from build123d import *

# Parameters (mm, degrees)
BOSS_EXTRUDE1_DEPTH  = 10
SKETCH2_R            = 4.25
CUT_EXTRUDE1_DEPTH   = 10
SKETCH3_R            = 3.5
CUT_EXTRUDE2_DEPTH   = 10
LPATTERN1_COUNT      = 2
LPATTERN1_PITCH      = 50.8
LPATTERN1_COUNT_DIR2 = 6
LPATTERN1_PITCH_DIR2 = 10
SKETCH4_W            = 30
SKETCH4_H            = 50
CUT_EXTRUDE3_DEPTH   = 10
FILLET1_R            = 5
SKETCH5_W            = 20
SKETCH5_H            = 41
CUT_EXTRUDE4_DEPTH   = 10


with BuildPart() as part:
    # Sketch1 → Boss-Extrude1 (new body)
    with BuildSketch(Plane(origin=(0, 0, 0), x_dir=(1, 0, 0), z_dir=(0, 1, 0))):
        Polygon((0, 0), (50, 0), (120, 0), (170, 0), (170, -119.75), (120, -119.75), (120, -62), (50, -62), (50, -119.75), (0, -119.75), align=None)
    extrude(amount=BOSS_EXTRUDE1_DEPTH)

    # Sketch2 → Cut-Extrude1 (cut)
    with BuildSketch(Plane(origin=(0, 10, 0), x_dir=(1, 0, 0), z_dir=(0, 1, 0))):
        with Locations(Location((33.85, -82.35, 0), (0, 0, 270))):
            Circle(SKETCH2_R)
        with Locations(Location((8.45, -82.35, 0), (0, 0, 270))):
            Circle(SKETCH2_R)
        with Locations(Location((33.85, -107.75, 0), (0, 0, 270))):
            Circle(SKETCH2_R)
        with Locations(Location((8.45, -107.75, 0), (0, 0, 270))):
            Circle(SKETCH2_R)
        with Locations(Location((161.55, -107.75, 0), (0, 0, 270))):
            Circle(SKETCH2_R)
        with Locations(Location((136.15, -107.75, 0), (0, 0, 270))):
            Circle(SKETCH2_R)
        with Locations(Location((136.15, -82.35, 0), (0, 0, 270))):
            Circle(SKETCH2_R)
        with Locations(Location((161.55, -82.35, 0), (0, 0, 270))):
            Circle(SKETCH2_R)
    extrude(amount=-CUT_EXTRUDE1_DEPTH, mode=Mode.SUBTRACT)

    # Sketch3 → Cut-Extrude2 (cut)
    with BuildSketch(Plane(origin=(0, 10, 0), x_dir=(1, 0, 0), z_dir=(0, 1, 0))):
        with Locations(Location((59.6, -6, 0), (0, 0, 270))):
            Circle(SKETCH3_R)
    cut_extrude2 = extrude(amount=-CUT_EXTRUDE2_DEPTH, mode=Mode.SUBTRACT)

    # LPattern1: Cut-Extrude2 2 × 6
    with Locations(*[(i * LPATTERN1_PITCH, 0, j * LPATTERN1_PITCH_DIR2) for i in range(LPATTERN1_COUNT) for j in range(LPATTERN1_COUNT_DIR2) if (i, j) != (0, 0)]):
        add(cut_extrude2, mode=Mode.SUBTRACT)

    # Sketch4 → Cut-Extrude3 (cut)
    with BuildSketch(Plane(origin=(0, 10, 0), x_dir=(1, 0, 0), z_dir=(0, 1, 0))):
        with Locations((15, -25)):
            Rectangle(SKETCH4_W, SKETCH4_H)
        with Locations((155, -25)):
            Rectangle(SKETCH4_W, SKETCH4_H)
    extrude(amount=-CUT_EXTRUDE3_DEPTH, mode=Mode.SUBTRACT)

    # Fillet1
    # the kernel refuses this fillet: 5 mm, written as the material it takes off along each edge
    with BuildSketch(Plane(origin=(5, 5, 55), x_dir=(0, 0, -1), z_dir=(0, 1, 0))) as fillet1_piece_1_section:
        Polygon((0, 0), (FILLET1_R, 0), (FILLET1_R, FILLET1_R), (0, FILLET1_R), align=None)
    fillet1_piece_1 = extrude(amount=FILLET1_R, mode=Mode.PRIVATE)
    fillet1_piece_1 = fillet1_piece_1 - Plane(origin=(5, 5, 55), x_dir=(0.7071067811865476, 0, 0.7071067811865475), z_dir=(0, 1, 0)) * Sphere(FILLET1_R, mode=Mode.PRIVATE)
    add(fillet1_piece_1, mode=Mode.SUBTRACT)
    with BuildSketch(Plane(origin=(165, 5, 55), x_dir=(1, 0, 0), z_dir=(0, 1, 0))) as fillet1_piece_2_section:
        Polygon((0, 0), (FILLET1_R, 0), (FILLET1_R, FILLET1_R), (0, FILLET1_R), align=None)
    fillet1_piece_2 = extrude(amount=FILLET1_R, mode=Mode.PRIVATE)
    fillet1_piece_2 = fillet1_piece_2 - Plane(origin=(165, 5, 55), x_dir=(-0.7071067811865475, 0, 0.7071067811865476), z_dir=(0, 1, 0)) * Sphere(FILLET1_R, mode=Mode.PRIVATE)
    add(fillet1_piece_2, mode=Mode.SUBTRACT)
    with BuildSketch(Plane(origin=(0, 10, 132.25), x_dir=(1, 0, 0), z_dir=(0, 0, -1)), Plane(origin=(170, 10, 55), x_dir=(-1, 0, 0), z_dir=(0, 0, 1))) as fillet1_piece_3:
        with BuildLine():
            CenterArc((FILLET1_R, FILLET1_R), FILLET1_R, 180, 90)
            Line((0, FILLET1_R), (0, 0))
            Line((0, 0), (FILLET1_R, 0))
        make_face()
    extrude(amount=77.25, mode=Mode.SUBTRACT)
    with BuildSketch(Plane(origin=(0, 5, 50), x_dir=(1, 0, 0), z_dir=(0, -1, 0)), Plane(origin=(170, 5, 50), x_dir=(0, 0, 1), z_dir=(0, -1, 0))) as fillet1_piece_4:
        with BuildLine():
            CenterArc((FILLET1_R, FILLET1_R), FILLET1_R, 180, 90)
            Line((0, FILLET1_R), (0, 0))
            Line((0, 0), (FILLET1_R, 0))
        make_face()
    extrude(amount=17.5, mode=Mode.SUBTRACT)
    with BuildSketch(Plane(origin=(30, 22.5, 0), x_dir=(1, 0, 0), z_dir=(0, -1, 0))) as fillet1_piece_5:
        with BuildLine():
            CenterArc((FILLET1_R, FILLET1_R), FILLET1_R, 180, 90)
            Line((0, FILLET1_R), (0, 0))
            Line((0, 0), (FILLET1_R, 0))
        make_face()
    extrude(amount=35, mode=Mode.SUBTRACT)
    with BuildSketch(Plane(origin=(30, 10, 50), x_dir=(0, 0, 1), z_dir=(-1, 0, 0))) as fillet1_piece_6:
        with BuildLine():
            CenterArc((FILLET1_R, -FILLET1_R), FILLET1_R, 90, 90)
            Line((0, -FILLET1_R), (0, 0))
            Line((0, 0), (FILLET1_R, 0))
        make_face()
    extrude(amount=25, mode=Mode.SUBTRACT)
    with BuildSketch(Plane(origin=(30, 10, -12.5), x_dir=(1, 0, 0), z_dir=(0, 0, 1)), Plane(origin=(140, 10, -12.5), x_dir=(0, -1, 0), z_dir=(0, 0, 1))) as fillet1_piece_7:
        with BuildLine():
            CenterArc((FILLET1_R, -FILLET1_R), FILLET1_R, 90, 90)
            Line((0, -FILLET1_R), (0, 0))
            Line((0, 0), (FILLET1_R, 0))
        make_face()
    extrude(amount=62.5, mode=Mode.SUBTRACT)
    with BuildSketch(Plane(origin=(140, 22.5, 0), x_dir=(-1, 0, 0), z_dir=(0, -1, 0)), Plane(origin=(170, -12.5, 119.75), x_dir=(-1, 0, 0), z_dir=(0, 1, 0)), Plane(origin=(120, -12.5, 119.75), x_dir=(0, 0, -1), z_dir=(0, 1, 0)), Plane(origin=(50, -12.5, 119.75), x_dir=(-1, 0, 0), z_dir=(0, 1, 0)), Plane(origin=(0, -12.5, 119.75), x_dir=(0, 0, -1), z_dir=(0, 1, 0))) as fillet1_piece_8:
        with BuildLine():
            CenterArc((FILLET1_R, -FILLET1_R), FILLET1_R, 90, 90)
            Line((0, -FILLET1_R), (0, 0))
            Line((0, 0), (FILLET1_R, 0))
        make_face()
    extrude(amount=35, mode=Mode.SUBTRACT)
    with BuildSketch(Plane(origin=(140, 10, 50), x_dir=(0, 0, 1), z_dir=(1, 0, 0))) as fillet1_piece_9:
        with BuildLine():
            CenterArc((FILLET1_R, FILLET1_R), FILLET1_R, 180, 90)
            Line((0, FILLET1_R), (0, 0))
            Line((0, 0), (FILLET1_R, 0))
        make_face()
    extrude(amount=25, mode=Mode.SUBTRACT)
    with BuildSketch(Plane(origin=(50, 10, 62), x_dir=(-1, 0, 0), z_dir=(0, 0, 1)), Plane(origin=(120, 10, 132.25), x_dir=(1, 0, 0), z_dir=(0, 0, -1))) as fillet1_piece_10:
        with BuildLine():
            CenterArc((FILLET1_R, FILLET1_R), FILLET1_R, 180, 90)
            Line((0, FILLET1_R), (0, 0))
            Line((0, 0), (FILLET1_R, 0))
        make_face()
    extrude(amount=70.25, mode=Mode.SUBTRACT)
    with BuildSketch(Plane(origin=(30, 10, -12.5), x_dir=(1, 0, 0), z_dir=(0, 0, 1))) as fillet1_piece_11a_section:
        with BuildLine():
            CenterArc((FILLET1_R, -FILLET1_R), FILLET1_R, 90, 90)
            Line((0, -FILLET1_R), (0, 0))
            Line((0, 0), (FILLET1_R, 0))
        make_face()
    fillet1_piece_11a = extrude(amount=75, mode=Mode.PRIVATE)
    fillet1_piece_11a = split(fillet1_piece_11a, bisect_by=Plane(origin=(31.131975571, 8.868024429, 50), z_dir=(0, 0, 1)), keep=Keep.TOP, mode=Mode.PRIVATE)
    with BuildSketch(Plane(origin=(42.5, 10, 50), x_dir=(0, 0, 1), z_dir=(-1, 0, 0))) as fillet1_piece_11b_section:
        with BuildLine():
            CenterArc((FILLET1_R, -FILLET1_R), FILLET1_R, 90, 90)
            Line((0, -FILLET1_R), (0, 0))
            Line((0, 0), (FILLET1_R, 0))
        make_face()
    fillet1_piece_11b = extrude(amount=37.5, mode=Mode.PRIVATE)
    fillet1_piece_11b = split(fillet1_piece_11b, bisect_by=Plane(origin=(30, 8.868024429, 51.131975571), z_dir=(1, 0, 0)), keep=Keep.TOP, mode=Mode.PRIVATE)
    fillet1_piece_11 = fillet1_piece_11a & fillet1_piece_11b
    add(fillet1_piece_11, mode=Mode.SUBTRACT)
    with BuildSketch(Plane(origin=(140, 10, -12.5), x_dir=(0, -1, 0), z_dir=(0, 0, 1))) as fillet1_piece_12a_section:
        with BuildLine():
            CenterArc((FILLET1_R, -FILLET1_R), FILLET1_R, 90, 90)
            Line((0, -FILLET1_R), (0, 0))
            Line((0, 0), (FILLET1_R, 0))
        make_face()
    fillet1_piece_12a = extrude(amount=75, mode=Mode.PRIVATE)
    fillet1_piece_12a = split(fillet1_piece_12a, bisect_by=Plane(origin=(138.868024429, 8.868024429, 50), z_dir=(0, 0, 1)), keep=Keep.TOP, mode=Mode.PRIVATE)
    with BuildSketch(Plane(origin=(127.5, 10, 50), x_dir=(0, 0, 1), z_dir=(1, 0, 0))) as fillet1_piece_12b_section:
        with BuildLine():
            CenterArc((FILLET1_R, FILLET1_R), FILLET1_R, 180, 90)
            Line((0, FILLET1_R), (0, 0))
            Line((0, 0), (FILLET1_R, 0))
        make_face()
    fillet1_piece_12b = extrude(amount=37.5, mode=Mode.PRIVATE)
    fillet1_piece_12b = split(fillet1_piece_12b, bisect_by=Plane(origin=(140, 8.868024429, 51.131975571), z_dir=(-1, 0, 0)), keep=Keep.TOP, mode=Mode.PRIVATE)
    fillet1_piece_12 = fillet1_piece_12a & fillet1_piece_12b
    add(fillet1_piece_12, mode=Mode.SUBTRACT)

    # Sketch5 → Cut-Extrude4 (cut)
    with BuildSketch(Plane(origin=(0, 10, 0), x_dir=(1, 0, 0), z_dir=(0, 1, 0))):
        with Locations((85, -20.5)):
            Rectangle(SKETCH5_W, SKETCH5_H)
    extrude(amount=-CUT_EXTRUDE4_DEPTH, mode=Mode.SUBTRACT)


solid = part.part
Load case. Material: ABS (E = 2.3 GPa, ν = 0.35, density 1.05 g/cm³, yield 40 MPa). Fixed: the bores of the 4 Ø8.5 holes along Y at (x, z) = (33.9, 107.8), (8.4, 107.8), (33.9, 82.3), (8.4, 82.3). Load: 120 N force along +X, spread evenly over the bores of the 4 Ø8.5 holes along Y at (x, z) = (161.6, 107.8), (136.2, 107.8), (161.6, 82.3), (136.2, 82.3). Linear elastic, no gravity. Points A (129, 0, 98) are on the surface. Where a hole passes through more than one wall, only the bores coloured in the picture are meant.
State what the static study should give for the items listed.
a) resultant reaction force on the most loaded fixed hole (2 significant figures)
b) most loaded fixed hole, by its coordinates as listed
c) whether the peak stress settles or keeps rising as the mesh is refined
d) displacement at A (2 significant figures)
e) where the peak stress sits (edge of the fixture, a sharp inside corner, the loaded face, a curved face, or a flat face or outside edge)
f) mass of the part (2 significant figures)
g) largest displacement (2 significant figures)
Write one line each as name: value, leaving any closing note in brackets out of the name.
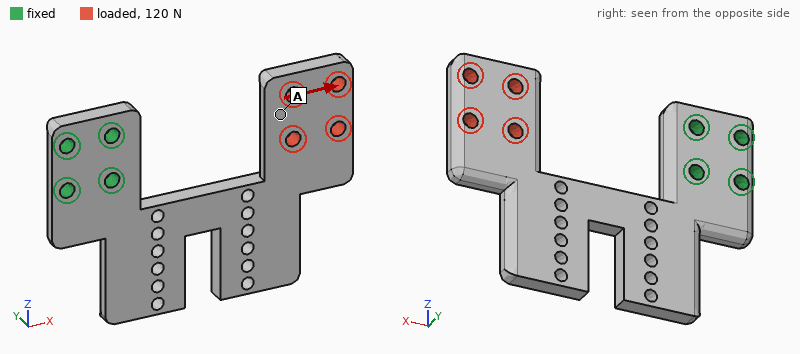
resultant reaction force on the most loaded fixed hole: 130 N
most loaded fixed hole, by its coordinates as listed: (33.9, 82.3)
whether the peak stress settles or keeps rising as the mesh is refined: keeps rising
displacement at A: 1.5 mm
where the peak stress sits: a sharp inside corner
mass of the part: 120 g
largest displacement: 2.5 mm
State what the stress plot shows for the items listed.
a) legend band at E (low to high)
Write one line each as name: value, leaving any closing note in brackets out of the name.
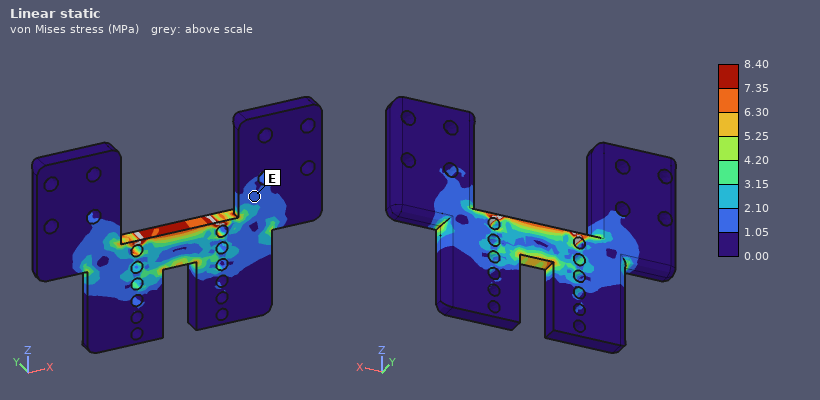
legend band at E: 1.05 to 2.10 MPa
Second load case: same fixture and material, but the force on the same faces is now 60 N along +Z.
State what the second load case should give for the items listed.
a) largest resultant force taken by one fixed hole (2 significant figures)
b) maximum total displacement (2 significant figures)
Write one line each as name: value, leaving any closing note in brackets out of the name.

largest resultant force taken by one fixed hole: 220 N
maximum total displacement: 2.1 mm
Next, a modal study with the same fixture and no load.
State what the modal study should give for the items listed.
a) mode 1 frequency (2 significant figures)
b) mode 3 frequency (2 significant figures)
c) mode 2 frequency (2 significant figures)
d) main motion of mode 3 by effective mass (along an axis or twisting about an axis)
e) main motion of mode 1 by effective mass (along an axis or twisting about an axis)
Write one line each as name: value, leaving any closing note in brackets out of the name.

mode 1 frequency: 65 Hz
mode 3 frequency: 150 Hz
mode 2 frequency: 140 Hz
main motion of mode 3 by effective mass: along Z
main motion of mode 1 by effective mass: along Y
